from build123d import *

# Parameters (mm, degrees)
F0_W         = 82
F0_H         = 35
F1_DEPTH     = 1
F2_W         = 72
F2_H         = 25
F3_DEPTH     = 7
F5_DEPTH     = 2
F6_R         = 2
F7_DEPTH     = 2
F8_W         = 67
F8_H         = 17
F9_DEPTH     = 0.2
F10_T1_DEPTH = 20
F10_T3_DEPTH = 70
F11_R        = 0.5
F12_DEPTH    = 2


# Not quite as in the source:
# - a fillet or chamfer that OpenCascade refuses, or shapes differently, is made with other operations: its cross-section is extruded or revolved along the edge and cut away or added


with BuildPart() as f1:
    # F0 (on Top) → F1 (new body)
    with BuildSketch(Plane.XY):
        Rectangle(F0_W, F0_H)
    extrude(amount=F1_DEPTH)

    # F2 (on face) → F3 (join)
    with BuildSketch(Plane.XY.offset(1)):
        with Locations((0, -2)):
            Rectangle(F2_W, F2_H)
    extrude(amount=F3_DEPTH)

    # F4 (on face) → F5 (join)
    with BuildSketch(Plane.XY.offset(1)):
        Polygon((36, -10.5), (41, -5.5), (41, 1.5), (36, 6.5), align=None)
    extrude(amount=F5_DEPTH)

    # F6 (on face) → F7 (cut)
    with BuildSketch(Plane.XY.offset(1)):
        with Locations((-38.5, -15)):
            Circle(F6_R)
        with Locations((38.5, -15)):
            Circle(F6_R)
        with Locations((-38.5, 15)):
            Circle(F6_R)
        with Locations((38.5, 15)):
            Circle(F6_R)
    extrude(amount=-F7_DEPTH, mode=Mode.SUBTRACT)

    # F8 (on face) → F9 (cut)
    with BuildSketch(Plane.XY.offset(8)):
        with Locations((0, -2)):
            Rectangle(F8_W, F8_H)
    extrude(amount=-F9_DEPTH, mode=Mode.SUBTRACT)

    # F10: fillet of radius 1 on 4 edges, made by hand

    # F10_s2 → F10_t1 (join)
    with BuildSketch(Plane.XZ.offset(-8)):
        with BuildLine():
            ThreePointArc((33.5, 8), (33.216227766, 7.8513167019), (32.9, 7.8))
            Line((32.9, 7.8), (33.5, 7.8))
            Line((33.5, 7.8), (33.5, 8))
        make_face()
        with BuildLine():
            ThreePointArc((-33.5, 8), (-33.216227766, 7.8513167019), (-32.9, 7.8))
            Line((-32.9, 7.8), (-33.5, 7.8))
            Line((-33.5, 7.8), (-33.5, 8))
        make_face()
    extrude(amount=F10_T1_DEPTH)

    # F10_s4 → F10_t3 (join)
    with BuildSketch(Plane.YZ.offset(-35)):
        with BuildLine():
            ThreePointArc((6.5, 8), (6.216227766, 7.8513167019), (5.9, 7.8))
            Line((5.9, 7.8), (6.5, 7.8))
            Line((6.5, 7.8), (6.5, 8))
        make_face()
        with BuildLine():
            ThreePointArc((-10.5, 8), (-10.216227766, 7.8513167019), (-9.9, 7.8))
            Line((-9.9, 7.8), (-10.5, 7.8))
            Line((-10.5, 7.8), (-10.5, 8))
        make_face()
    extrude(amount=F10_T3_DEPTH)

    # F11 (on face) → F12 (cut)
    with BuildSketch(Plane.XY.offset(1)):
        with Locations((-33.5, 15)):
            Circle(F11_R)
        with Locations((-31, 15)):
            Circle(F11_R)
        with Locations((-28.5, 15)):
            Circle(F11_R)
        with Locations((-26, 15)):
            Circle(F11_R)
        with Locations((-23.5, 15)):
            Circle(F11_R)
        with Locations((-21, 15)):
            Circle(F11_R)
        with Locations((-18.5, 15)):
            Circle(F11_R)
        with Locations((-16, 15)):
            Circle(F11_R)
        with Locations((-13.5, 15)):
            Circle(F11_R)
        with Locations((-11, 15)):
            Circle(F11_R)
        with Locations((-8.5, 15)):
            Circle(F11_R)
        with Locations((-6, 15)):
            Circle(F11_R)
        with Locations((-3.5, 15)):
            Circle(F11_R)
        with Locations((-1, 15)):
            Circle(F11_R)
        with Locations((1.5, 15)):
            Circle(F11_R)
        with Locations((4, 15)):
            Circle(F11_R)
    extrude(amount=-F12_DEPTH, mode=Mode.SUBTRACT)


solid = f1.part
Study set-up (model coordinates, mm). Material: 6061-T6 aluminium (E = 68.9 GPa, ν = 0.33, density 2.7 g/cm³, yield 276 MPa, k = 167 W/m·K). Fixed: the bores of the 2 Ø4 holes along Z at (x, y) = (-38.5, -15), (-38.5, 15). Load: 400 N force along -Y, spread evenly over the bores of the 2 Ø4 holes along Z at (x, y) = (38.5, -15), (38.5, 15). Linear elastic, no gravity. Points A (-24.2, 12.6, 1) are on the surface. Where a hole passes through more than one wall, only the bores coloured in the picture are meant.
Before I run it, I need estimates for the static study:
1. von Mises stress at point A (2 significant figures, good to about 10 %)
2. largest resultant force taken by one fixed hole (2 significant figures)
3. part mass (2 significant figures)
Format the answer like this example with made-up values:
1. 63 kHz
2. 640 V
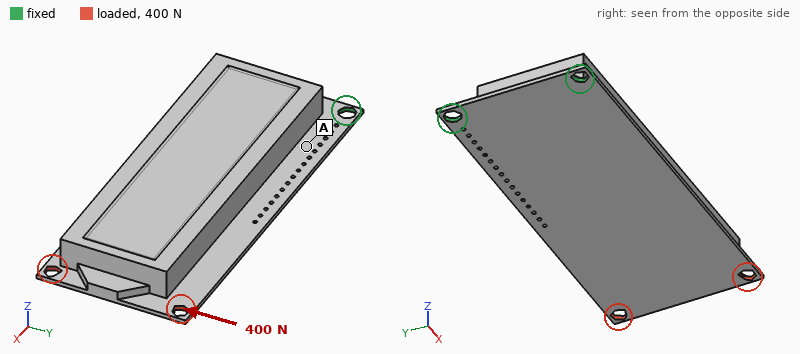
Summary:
1. 54 MPa
2. 1.1 kN
3. 41 g
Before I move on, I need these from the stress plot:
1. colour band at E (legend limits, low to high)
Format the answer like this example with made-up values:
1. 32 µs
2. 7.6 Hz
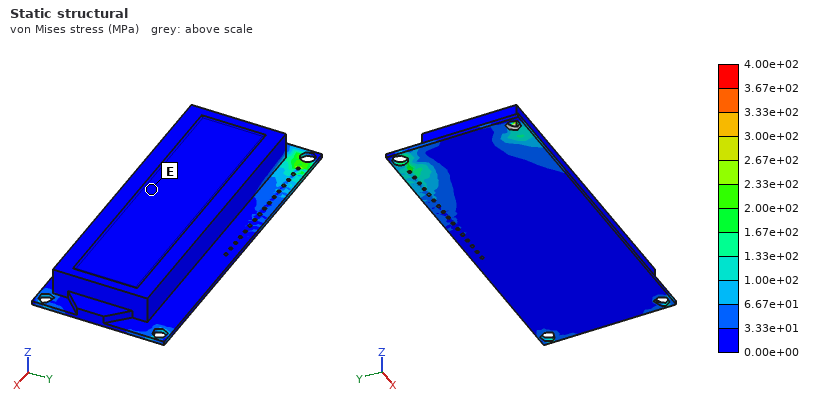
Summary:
1. 0.00e+00 to 3.33e+01 MPa
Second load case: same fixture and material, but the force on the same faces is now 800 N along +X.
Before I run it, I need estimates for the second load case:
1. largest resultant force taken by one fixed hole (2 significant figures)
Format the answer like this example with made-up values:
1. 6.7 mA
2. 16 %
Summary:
1. 430 N
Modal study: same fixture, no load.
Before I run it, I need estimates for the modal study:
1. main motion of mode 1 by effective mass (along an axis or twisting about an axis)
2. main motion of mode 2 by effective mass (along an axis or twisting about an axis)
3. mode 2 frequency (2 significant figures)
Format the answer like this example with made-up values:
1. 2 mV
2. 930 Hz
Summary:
1. along Z
2. along Y
3. 2500 Hz
